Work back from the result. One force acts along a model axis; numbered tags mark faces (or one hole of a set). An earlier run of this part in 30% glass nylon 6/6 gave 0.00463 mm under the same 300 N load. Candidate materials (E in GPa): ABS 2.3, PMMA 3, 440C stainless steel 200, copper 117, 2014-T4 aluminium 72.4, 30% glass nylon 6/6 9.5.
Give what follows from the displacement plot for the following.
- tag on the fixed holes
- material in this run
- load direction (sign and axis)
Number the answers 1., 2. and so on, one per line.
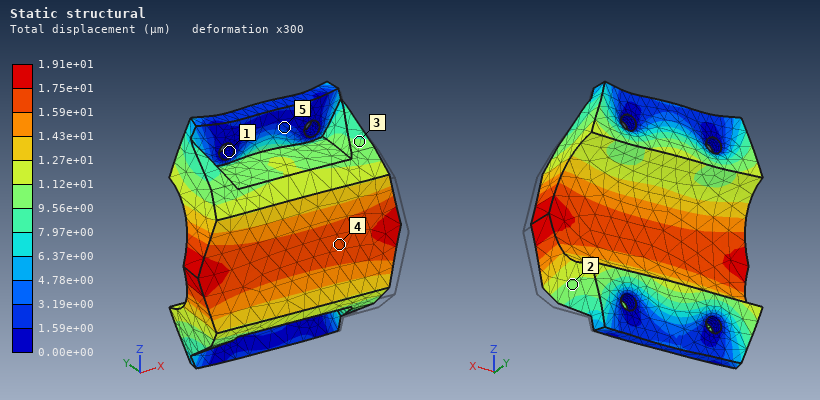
1. 1
2. ABS
3. +Y
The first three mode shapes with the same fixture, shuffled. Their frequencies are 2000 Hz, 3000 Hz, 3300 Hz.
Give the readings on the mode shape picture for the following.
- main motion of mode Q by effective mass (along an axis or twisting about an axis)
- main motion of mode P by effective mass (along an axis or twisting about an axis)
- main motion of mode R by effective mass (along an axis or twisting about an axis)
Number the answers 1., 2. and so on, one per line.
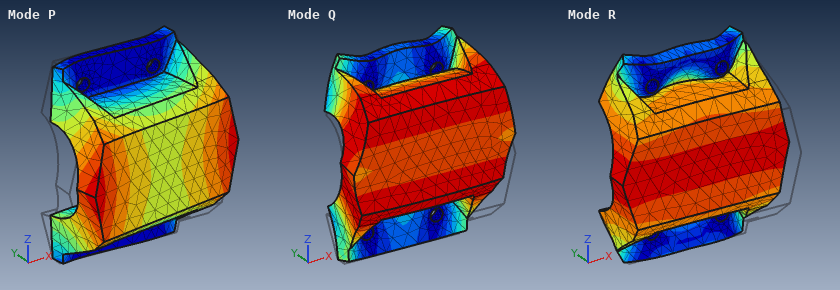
1. along Z
2. along X
3. along Y
